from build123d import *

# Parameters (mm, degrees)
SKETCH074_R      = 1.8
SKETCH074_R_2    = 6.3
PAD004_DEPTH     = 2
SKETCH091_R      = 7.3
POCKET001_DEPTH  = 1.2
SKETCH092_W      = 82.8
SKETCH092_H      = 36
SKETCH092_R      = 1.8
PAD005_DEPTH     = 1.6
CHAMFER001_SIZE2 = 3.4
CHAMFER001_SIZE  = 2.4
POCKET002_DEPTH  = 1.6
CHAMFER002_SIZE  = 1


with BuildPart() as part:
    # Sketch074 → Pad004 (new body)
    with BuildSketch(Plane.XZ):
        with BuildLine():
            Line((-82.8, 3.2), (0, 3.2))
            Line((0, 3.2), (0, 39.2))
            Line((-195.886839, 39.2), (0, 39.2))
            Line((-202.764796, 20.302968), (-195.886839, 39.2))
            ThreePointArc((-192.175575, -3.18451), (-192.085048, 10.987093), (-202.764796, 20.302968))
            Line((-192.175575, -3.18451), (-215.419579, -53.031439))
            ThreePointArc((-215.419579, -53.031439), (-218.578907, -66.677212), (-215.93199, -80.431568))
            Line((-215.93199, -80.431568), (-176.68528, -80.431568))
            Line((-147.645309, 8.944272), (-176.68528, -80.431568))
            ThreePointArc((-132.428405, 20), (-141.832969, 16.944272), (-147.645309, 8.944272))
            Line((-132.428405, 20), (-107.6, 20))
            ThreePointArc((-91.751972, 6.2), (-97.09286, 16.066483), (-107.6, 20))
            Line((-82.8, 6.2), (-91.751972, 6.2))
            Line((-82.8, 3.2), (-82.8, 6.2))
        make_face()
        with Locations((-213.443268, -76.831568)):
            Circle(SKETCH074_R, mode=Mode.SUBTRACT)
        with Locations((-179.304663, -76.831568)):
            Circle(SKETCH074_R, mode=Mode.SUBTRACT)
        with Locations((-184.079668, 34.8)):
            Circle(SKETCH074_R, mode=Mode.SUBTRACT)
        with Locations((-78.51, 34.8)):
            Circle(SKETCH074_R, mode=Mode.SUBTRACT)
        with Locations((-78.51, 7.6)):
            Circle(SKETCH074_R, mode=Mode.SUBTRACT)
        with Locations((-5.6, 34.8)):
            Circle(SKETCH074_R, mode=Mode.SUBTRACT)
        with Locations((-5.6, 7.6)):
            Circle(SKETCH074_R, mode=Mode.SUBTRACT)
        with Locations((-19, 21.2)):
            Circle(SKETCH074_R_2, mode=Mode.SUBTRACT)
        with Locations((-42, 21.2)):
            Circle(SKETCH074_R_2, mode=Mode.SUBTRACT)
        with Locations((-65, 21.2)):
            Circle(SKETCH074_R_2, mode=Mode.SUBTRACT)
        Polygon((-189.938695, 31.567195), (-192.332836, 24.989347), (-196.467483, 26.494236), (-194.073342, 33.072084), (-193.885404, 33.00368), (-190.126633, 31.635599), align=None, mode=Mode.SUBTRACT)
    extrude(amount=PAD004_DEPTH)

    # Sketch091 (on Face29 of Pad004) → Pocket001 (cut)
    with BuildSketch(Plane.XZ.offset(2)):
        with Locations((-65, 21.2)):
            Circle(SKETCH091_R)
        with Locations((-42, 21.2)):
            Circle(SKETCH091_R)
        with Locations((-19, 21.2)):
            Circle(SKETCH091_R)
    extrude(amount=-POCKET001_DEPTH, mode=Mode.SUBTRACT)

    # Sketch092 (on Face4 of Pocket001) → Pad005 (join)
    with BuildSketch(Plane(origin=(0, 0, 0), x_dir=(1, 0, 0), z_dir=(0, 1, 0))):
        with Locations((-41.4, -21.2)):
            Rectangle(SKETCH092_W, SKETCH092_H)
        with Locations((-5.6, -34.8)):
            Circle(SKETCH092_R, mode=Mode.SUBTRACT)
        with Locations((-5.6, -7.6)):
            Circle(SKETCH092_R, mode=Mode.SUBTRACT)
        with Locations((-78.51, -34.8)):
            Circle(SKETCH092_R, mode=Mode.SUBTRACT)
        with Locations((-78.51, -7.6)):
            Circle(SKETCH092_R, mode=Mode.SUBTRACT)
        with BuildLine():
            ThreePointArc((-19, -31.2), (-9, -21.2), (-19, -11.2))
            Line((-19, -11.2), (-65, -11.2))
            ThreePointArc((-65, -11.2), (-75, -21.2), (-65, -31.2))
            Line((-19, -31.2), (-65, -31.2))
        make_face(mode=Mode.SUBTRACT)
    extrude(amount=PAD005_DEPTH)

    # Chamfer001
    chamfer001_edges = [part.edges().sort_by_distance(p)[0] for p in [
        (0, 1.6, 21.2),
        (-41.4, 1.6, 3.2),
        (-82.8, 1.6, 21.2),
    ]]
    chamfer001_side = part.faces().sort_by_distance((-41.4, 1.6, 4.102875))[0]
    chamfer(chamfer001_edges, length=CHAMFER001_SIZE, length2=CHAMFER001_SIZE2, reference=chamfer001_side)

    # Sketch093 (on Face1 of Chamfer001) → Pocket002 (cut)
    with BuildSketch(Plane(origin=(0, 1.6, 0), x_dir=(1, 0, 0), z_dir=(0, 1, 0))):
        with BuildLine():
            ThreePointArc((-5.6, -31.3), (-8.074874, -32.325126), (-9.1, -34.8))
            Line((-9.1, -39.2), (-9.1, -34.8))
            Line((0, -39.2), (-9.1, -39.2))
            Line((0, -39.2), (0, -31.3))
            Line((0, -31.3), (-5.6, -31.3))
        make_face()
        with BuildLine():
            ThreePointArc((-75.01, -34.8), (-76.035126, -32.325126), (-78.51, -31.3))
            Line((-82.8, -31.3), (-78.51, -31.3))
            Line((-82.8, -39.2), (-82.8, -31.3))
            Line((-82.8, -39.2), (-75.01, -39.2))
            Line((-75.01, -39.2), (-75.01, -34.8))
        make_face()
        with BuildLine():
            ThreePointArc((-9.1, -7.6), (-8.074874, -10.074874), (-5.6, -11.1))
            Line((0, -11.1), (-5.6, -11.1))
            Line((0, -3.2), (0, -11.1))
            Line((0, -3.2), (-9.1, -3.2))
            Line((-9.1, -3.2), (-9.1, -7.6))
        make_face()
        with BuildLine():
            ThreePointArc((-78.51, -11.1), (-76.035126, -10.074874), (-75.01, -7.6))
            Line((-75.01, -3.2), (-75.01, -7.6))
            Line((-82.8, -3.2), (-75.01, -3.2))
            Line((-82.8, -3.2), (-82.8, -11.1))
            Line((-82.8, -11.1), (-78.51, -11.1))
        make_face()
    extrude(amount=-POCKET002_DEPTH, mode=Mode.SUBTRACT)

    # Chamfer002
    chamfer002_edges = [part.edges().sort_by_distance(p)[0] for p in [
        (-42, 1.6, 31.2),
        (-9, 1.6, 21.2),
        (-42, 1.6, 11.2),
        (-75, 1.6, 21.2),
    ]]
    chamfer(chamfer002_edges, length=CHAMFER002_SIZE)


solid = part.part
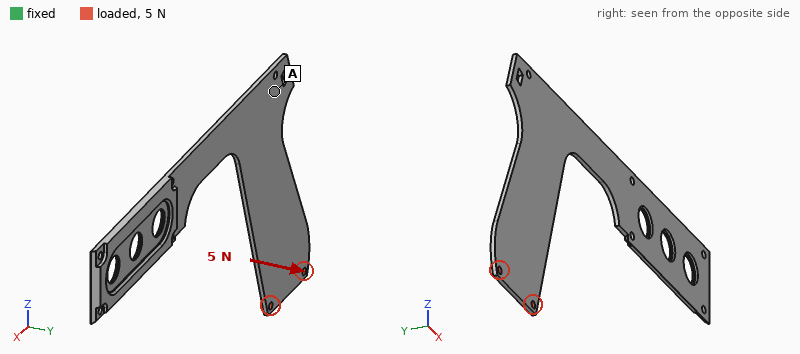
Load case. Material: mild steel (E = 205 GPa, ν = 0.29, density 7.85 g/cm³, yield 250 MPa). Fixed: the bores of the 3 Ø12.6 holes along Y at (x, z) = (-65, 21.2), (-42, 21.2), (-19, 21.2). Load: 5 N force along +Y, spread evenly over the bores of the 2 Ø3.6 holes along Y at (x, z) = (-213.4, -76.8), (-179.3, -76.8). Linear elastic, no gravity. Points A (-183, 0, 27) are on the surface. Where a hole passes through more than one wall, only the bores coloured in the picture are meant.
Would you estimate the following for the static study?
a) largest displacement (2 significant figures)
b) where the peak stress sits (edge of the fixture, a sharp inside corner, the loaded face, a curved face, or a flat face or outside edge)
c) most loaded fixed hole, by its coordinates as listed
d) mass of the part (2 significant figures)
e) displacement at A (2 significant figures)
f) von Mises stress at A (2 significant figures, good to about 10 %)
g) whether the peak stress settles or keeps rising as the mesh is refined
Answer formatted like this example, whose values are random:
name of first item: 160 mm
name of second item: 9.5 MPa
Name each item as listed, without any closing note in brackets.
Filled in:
largest displacement: 2.5 mm
where the peak stress sits: edge of the fixture
most loaded fixed hole, by its coordinates as listed: (-65, 21.2)
mass of the part: 160 g
displacement at A: 0.75 mm
von Mises stress at A: 8.2 MPa
whether the peak stress settles or keeps rising as the mesh is refined: keeps rising
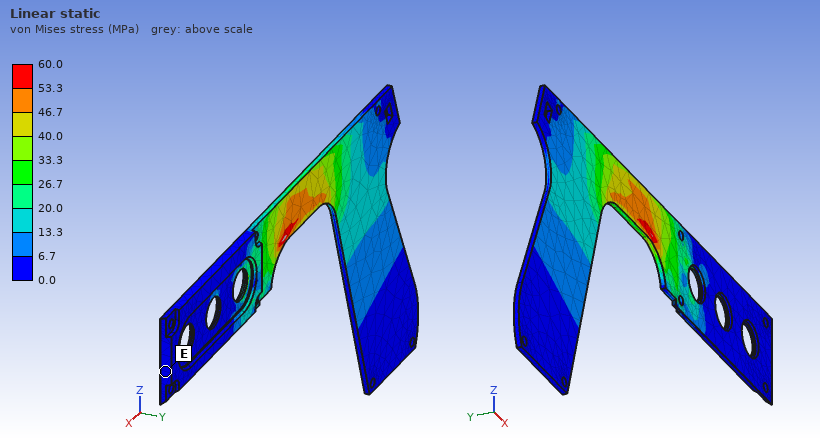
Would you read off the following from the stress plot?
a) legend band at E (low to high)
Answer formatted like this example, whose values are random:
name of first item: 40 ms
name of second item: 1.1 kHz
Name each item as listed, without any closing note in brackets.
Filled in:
legend band at E: 0.0 to 6.7 MPa
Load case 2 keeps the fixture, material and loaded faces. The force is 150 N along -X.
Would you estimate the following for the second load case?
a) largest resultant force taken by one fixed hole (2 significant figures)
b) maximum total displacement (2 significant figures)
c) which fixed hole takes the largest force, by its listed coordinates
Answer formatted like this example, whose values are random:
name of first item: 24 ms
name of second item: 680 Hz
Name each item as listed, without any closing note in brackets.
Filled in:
largest resultant force taken by one fixed hole: 300 N
maximum total displacement: 0.63 mm
which fixed hole takes the largest force, by its listed coordinates: (-65, 21.2)
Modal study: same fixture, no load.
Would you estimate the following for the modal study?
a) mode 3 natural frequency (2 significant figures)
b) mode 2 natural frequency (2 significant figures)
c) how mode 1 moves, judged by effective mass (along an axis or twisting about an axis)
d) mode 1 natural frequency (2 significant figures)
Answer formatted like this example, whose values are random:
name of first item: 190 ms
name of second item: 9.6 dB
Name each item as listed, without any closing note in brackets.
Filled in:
mode 3 natural frequency: 370 Hz
mode 2 natural frequency: 130 Hz
how mode 1 moves, judged by effective mass: along Y
mode 1 natural frequency: 39 Hz
